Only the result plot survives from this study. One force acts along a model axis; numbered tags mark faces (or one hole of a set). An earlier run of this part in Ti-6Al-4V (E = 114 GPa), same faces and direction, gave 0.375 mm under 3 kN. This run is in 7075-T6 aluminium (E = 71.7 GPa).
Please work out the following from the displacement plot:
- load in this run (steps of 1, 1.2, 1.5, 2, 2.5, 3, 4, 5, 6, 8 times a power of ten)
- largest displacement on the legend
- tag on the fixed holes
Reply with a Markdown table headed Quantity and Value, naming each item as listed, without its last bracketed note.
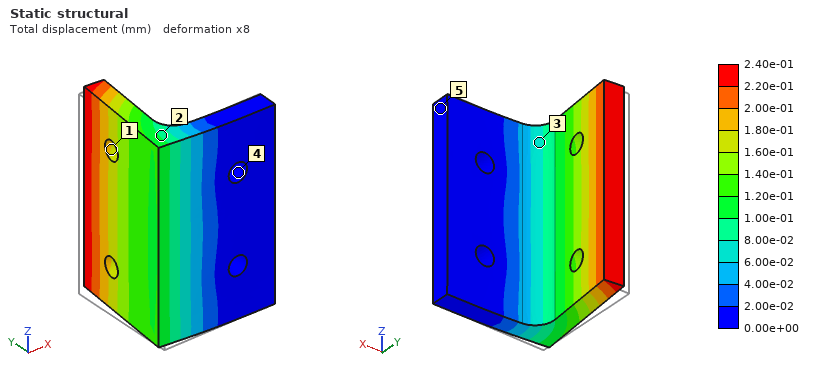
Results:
| Quantity | Value |
|---|---|
| load in this run | 1.2 kN |
| largest displacement on the legend | 2.40e-01 mm |
| tag on the fixed holes | 4 |
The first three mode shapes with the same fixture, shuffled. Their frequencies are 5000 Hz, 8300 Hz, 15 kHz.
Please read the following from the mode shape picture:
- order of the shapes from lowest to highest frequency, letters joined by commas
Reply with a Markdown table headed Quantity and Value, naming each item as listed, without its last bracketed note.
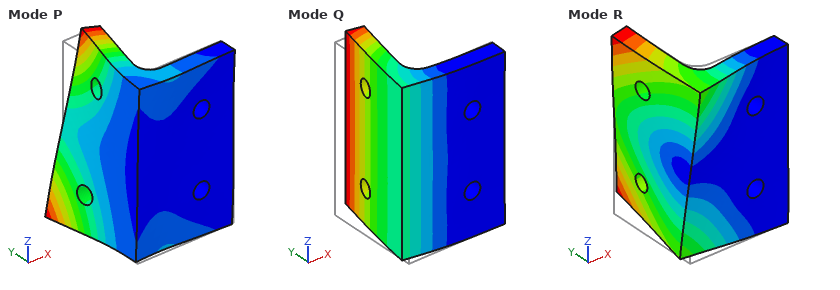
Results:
| Quantity | Value |
|---|---|
| order of the shapes from lowest to highest frequency, letters joined by commas | Q, R, P |
